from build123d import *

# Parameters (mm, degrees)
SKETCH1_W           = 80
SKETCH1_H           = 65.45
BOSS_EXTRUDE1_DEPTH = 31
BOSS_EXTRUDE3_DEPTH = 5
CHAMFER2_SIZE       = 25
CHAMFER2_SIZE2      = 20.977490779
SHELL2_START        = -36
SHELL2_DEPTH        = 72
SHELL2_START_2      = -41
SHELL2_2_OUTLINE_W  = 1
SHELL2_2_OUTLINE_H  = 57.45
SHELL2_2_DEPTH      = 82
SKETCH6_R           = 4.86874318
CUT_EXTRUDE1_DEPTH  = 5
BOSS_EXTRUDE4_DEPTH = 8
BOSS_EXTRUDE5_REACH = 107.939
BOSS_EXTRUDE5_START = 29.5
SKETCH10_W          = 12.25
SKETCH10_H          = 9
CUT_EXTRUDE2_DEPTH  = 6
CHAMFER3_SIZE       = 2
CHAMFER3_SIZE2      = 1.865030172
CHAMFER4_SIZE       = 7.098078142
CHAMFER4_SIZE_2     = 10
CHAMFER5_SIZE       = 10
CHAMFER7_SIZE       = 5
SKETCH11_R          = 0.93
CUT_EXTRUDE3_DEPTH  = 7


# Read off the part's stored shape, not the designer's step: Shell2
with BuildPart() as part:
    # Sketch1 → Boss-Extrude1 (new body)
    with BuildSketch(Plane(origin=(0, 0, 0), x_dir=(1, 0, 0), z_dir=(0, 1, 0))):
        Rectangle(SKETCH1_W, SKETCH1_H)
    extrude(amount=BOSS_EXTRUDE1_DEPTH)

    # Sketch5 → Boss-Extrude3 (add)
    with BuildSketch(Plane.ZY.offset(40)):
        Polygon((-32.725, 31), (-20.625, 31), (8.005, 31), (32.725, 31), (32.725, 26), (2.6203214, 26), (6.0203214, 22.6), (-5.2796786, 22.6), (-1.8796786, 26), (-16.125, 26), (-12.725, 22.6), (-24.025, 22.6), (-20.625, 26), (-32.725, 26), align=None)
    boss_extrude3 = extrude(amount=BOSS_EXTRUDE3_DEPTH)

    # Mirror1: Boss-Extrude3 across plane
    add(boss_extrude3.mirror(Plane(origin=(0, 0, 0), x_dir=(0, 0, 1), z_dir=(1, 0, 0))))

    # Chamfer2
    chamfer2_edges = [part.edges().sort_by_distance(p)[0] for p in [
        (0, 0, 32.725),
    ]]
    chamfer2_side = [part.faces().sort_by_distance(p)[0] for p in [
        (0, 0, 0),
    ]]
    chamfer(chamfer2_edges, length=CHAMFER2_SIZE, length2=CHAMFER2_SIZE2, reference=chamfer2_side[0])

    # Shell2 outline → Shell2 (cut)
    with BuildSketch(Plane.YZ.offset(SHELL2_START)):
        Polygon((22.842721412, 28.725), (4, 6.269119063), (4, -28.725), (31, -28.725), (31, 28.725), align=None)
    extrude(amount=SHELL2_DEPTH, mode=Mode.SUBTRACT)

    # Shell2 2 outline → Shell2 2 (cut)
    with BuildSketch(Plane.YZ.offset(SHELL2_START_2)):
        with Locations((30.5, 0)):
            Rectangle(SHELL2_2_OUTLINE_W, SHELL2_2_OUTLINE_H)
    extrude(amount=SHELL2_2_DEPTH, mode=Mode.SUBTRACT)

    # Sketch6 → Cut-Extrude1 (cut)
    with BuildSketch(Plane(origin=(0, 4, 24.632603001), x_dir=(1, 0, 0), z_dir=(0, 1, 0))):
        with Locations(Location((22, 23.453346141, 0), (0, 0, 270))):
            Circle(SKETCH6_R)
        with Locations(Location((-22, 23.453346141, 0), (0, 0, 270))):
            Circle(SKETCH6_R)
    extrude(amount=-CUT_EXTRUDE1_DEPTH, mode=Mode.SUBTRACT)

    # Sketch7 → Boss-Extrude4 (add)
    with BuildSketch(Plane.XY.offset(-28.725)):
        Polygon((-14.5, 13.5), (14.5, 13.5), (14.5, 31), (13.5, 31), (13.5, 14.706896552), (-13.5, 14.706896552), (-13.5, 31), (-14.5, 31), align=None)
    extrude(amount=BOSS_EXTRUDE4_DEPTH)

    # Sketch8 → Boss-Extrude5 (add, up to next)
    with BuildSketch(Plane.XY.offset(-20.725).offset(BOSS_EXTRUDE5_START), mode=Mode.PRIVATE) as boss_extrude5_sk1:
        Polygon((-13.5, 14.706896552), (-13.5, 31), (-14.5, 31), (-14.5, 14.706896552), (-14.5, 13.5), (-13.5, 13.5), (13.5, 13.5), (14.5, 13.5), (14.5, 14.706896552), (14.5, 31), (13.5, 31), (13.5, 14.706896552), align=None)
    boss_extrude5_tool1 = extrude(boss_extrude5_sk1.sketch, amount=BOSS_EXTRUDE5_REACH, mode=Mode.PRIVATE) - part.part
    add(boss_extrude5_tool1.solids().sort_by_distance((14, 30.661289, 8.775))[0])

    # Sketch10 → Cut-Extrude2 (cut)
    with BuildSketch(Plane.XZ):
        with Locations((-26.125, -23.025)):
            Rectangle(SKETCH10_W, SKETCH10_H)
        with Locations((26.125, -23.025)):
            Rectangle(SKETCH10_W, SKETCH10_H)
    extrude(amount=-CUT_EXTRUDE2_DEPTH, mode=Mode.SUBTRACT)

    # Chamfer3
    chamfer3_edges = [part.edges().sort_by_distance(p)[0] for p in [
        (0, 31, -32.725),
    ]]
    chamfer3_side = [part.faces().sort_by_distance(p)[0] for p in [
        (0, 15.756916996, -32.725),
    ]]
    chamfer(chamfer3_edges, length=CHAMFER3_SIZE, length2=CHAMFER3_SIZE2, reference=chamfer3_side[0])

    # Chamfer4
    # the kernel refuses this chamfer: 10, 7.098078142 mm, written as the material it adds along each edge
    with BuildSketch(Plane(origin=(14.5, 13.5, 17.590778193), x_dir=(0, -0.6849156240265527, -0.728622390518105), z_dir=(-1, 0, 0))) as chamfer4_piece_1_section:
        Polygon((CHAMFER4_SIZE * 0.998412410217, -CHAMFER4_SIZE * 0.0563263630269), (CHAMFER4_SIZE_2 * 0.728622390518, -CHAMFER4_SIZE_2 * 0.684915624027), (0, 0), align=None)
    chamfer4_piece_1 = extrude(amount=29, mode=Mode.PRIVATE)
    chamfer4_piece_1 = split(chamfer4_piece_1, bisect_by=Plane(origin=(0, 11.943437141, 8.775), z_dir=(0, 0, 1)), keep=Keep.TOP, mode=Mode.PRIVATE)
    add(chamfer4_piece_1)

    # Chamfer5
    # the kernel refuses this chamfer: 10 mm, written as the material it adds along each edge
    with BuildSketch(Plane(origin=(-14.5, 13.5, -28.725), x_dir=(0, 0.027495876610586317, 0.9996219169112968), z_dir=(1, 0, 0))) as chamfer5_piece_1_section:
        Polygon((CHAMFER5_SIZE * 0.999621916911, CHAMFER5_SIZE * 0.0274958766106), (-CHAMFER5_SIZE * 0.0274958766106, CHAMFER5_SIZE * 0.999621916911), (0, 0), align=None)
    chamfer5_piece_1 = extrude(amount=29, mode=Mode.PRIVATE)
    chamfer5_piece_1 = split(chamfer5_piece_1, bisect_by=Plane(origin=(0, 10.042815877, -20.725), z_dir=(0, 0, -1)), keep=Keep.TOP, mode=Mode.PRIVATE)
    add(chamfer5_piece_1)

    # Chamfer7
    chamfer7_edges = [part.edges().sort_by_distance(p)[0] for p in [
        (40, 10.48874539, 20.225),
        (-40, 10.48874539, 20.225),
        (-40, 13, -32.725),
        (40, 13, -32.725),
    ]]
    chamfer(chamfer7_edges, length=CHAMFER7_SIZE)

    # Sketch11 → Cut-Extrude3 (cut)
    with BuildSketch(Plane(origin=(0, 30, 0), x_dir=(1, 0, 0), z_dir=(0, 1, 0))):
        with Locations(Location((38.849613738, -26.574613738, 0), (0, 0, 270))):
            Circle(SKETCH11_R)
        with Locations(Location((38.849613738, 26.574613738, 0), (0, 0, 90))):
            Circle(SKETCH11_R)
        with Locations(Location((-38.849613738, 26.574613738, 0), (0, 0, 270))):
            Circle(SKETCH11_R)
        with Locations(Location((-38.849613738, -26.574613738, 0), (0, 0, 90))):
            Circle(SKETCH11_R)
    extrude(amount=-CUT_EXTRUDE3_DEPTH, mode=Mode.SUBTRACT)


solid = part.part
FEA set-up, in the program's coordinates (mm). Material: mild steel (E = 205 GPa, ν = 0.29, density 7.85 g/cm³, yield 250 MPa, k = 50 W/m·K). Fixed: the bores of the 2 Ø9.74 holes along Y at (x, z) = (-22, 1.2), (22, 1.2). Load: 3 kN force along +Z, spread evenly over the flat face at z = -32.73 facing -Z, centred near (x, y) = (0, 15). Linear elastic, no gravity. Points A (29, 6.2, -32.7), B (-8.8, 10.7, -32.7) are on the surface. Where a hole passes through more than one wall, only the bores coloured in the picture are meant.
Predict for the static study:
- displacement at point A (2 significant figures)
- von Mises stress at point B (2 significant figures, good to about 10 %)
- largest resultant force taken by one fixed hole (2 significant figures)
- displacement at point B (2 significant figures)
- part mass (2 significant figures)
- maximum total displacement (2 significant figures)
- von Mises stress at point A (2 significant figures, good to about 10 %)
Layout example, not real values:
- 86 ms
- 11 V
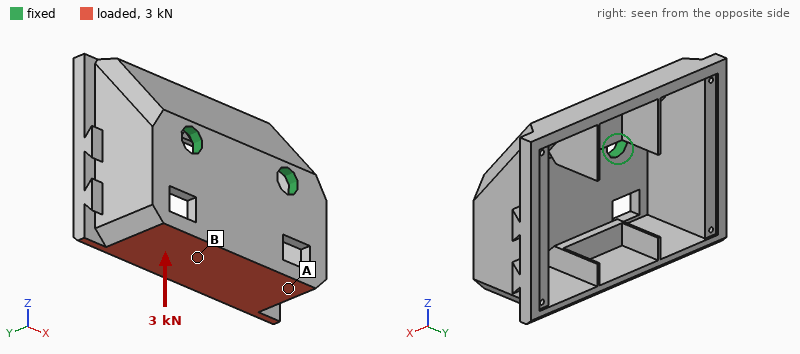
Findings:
- 0.062 mm
- 23 MPa
- 1.5 kN
- 0.072 mm
- 380 g
- 0.14 mm
- 60 MPa
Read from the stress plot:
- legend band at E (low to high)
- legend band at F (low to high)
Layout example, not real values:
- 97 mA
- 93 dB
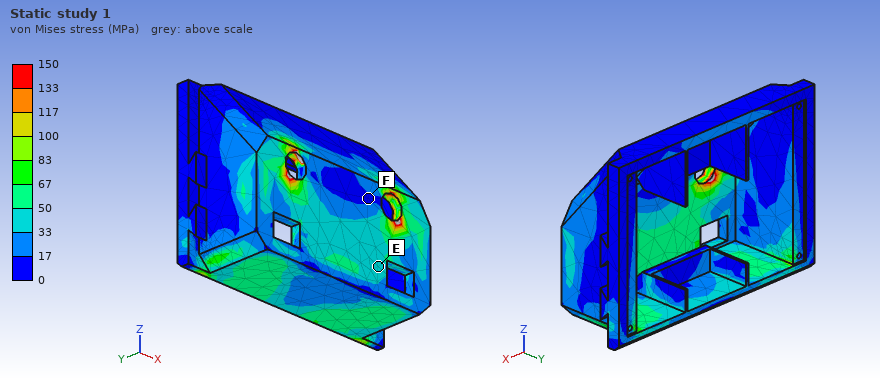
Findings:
- 33 to 50 MPa
- 0 to 17 MPa
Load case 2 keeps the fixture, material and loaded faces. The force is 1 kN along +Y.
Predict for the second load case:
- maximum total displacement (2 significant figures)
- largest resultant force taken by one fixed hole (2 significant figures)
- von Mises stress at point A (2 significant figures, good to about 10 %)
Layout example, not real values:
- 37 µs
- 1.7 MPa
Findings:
- 70 µm
- 500 N
- 18 MPa
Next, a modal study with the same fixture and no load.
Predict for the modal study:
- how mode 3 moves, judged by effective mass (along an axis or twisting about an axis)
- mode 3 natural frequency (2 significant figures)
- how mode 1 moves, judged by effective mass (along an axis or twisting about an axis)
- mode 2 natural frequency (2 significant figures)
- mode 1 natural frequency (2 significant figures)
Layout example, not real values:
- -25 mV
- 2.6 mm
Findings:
- along Y
- 4000 Hz
- along Z
- 2300 Hz
- 1600 Hz
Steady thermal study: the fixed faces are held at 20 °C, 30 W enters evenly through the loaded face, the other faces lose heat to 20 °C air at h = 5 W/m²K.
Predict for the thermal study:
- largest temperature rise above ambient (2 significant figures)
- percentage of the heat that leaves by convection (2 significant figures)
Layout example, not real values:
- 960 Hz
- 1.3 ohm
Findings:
- 62 K
- 9.6 %
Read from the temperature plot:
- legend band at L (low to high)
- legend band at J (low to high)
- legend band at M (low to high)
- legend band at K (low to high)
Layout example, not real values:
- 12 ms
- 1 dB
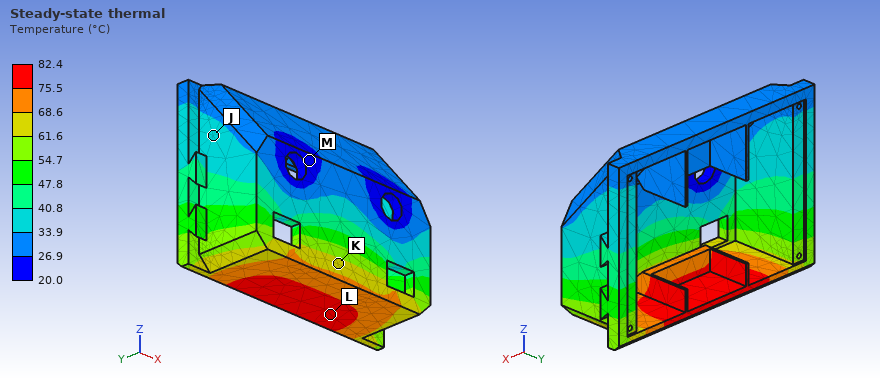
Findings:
- 75.5 to 82.4 °C
- 33.9 to 40.8 °C
- 20.0 to 26.9 °C
- 61.6 to 68.6 °C
